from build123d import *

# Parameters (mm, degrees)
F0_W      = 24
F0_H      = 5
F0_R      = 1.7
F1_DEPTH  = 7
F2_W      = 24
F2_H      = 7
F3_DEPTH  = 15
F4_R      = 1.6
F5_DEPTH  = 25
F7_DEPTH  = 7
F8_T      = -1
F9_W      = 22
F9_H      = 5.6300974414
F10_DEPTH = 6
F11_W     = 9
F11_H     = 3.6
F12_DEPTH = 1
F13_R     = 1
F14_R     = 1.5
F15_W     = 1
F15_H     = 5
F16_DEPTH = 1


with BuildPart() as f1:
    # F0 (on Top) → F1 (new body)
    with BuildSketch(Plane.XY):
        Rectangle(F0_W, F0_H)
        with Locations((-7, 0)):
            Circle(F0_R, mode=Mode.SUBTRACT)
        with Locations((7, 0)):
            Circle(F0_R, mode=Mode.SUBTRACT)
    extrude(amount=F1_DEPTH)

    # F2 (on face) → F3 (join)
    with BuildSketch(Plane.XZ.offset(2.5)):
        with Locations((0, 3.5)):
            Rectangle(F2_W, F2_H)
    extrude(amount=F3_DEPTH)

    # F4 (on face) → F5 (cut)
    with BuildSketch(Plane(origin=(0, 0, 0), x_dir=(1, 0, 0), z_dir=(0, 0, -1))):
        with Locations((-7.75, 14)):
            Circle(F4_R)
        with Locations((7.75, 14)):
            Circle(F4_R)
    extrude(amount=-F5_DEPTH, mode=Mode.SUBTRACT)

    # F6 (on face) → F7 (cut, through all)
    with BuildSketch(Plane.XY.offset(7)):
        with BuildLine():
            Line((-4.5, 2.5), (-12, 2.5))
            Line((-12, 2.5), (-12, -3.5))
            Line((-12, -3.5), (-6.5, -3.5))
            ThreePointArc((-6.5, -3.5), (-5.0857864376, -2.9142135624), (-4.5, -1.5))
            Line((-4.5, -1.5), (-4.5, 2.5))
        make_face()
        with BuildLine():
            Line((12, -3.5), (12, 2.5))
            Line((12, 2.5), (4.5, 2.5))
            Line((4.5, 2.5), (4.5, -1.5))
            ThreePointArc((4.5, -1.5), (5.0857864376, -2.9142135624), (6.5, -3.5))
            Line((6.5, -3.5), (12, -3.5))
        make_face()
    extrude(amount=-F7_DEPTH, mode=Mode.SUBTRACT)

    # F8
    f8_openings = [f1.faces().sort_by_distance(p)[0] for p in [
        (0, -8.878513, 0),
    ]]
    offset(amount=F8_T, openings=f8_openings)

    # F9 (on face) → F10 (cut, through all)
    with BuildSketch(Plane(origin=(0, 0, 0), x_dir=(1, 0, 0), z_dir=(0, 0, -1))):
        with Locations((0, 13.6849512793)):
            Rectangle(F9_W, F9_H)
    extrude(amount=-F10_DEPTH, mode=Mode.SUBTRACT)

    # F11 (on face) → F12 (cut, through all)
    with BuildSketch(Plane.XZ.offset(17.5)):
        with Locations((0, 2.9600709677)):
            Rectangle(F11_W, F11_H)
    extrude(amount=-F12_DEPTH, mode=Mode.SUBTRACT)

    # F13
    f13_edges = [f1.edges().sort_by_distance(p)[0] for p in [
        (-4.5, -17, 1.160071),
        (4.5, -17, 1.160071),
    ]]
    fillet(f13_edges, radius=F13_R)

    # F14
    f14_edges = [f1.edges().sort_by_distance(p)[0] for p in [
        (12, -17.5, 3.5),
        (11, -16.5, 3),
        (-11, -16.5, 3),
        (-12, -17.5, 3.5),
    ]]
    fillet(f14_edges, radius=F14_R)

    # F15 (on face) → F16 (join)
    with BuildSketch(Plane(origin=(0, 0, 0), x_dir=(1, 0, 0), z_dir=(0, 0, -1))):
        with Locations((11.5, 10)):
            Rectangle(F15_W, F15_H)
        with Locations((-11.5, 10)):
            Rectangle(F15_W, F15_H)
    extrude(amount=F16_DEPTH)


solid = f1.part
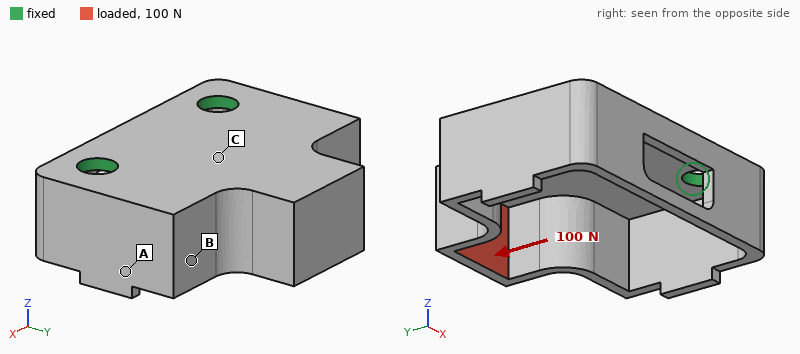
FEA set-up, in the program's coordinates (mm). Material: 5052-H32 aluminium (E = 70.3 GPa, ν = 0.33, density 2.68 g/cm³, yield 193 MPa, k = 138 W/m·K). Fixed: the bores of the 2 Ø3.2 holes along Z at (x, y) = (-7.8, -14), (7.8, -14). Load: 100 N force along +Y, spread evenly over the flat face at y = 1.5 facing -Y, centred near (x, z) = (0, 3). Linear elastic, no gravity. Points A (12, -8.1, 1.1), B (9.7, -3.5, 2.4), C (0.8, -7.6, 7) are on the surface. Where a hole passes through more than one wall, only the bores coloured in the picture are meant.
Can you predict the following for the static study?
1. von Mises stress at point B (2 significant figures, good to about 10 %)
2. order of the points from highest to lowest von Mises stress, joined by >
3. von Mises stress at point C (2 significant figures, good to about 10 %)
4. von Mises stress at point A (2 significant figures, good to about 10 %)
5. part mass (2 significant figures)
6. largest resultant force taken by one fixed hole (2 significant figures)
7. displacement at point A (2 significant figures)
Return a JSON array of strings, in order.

["57 MPa", "B > C > A", "22 MPa", "12 MPa", "2.3 g", "50 N", "0.017 mm"]
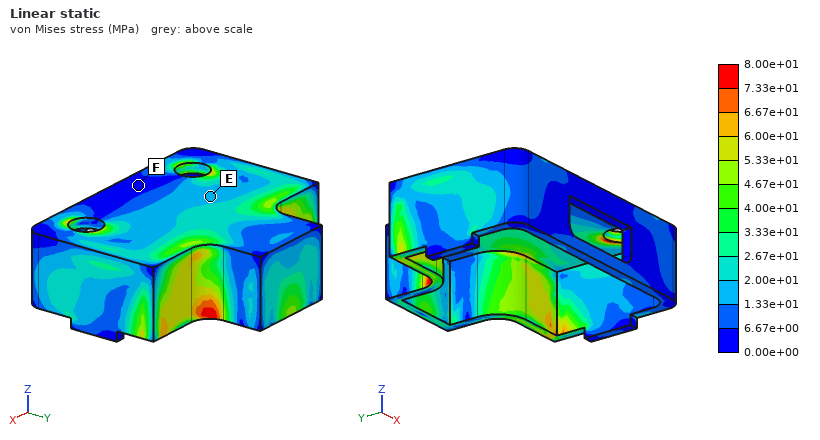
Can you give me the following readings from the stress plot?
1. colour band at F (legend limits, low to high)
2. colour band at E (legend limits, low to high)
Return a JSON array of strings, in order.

["0.00e+00 to 6.67e+00 MPa", "1.33e+01 to 2.00e+01 MPa"]
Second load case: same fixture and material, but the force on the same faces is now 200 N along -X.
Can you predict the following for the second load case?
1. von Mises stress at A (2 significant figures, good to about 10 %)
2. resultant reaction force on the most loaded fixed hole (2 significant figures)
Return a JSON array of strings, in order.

["22 MPa", "200 N"]
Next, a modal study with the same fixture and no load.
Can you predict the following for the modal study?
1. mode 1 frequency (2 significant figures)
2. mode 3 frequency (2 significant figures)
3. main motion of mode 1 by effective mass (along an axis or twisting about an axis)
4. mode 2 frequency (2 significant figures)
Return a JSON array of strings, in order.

["4500 Hz", "11 kHz", "along Z", "9200 Hz"]
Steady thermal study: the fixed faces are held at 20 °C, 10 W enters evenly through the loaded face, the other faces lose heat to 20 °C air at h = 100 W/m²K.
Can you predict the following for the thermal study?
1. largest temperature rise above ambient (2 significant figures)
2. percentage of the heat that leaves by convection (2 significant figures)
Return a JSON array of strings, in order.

["54 K", "24 %"]
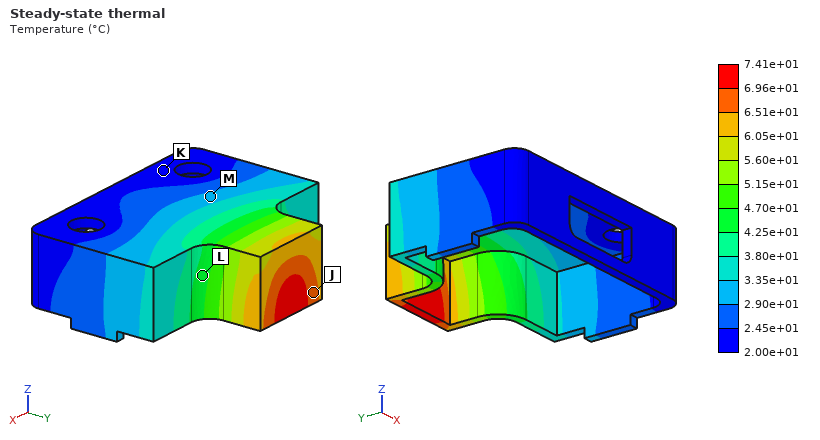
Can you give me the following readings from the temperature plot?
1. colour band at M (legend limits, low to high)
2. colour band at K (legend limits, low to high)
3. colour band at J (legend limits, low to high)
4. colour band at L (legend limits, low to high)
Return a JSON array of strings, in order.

["2.90e+01 to 3.35e+01 °C", "2.00e+01 to 2.45e+01 °C", "6.51e+01 to 6.96e+01 °C", "4.25e+01 to 4.70e+01 °C"]
